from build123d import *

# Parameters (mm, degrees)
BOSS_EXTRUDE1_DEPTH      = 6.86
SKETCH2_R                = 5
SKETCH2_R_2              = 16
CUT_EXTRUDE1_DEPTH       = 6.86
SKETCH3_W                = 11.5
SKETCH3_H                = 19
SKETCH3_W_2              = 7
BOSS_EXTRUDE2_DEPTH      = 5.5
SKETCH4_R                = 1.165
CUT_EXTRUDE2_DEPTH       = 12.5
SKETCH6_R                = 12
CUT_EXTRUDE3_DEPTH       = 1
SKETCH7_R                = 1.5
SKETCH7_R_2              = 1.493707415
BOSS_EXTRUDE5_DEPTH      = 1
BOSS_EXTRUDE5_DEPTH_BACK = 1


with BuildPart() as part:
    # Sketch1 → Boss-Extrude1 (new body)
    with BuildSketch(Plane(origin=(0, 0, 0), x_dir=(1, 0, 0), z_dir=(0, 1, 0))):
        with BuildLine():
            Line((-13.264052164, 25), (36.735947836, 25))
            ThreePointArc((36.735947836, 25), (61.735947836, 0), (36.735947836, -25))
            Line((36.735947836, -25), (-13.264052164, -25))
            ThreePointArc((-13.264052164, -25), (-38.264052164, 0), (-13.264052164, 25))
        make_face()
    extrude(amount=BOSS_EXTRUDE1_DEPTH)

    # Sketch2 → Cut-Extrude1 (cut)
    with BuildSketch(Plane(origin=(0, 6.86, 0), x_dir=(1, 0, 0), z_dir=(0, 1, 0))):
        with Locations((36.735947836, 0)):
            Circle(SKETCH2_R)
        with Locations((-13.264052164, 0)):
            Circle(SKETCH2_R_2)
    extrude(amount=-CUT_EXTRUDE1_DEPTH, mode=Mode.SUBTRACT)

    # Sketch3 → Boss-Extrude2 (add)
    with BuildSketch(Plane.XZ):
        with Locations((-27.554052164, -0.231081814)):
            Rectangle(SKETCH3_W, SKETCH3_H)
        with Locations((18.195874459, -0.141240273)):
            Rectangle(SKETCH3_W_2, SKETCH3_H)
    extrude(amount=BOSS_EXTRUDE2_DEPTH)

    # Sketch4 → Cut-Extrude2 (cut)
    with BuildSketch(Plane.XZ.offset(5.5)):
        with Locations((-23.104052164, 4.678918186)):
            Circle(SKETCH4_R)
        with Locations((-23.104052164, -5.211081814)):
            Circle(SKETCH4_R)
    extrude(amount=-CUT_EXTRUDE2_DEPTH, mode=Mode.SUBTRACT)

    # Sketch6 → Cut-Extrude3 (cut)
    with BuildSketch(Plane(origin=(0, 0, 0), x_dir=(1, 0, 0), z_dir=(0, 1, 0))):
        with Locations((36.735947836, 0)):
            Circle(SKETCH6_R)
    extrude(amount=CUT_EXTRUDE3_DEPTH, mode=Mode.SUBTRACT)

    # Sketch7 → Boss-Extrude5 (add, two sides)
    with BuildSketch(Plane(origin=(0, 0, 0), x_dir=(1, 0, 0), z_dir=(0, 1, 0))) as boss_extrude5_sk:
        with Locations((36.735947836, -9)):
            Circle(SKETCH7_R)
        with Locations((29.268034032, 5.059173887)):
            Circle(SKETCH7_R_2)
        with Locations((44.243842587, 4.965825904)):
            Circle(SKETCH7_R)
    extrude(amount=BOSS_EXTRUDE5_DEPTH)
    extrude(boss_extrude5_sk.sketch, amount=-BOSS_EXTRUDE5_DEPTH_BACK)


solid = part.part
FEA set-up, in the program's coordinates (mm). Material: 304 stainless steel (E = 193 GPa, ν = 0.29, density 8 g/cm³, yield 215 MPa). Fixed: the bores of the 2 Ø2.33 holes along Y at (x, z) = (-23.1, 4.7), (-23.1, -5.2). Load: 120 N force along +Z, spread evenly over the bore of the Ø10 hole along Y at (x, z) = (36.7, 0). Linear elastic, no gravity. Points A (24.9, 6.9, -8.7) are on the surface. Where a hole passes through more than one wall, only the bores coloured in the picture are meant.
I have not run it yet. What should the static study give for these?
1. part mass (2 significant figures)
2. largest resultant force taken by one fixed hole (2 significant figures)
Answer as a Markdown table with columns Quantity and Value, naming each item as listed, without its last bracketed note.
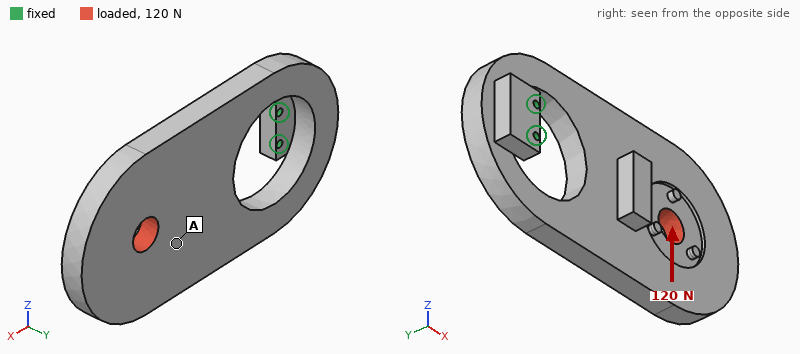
| Quantity | Value |
|---|---|
| part mass | 210 g |
| largest resultant force taken by one fixed hole | 640 N |
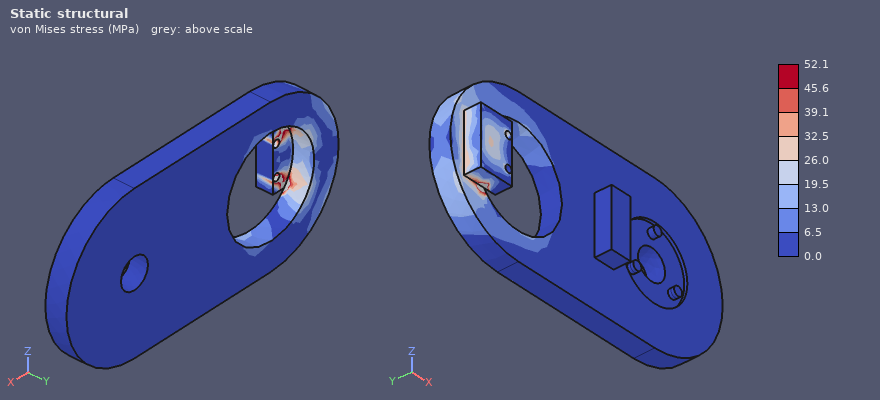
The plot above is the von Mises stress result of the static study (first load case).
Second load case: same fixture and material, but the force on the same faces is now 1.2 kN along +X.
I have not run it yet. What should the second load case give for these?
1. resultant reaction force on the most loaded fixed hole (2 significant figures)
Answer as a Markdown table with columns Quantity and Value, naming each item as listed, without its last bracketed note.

| Quantity | Value |
|---|---|
| resultant reaction force on the most loaded fixed hole | 650 N |
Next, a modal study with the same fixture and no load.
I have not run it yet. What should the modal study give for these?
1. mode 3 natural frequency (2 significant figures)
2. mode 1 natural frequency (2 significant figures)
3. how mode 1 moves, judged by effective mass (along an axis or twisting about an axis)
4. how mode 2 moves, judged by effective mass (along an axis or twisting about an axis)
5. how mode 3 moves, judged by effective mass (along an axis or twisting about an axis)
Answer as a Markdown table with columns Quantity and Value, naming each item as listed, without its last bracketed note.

| Quantity | Value |
|---|---|
| mode 3 natural frequency | 1700 Hz |
| mode 1 natural frequency | 310 Hz |
| how mode 1 moves, judged by effective mass | along Y |
| how mode 2 moves, judged by effective mass | along Z |
| how mode 3 moves, judged by effective mass | twisting about X |
